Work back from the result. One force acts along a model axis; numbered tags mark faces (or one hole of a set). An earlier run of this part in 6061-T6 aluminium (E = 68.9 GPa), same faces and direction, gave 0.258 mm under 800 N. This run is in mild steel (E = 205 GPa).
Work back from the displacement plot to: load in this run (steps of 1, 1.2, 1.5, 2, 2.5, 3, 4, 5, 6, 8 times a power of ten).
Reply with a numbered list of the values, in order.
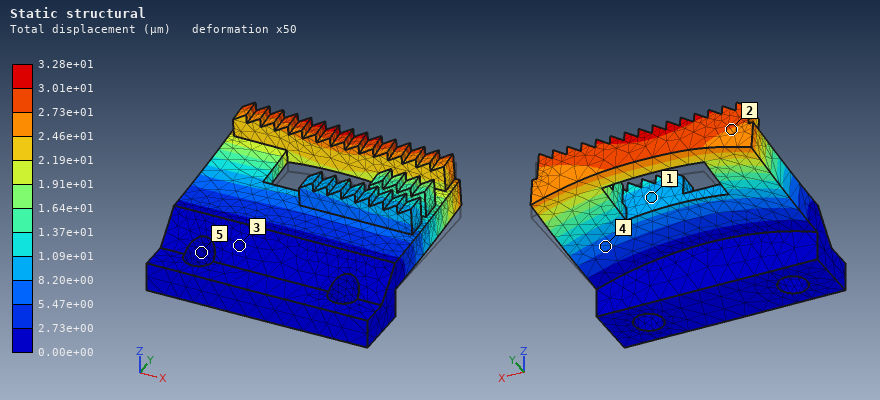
1. 300 N
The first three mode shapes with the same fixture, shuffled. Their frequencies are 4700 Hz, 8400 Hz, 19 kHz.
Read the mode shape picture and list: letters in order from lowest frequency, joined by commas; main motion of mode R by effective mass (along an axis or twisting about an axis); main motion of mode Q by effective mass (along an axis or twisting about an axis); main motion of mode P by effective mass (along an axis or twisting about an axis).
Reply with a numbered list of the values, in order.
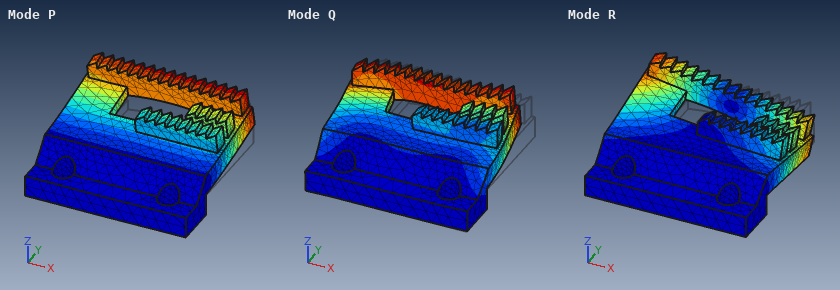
1. P, R, Q
2. twisting about Y
3. along X
4. along Z
